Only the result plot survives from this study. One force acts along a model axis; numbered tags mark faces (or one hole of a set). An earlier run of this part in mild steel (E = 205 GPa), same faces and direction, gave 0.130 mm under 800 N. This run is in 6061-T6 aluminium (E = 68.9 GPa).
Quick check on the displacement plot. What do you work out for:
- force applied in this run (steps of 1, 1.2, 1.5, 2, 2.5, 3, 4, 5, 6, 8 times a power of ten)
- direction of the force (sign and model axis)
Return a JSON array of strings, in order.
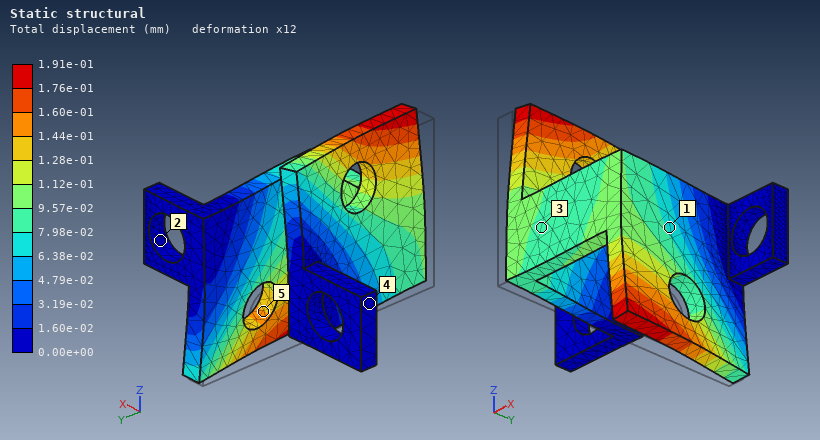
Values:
["400 N", "+X"]
